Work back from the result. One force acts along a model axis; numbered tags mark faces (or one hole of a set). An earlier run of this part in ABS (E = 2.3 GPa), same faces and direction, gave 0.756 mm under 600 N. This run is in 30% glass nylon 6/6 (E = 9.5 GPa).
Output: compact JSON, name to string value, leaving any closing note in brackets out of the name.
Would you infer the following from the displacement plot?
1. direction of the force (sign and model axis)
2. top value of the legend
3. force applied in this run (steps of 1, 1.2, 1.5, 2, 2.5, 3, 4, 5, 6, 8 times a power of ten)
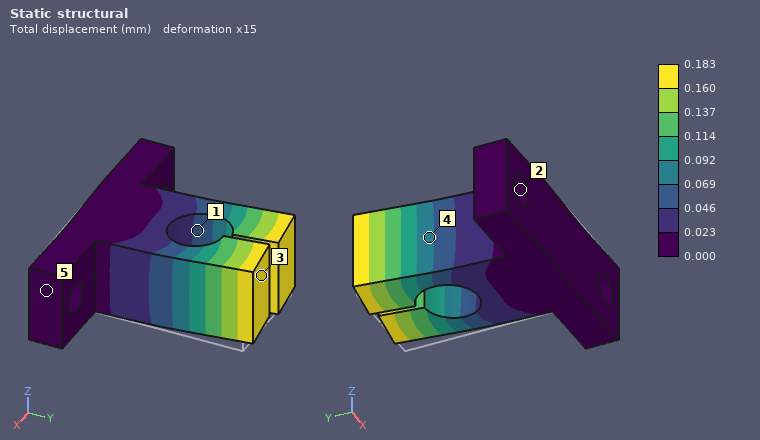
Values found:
{"direction of the force": "-X", "top value of the legend": "0.183 mm", "force applied in this run": "600 N"}
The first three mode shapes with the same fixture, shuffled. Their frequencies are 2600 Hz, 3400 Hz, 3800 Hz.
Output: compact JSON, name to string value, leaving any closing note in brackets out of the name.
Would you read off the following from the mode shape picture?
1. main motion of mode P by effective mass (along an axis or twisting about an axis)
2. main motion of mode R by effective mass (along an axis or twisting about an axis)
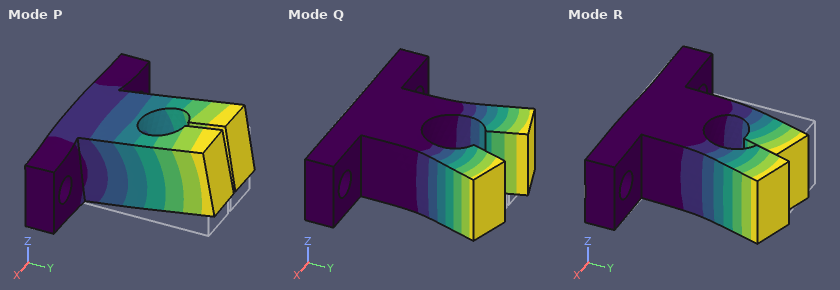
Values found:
{"main motion of mode P by effective mass": "along Z", "main motion of mode R by effective mass": "along X"}
